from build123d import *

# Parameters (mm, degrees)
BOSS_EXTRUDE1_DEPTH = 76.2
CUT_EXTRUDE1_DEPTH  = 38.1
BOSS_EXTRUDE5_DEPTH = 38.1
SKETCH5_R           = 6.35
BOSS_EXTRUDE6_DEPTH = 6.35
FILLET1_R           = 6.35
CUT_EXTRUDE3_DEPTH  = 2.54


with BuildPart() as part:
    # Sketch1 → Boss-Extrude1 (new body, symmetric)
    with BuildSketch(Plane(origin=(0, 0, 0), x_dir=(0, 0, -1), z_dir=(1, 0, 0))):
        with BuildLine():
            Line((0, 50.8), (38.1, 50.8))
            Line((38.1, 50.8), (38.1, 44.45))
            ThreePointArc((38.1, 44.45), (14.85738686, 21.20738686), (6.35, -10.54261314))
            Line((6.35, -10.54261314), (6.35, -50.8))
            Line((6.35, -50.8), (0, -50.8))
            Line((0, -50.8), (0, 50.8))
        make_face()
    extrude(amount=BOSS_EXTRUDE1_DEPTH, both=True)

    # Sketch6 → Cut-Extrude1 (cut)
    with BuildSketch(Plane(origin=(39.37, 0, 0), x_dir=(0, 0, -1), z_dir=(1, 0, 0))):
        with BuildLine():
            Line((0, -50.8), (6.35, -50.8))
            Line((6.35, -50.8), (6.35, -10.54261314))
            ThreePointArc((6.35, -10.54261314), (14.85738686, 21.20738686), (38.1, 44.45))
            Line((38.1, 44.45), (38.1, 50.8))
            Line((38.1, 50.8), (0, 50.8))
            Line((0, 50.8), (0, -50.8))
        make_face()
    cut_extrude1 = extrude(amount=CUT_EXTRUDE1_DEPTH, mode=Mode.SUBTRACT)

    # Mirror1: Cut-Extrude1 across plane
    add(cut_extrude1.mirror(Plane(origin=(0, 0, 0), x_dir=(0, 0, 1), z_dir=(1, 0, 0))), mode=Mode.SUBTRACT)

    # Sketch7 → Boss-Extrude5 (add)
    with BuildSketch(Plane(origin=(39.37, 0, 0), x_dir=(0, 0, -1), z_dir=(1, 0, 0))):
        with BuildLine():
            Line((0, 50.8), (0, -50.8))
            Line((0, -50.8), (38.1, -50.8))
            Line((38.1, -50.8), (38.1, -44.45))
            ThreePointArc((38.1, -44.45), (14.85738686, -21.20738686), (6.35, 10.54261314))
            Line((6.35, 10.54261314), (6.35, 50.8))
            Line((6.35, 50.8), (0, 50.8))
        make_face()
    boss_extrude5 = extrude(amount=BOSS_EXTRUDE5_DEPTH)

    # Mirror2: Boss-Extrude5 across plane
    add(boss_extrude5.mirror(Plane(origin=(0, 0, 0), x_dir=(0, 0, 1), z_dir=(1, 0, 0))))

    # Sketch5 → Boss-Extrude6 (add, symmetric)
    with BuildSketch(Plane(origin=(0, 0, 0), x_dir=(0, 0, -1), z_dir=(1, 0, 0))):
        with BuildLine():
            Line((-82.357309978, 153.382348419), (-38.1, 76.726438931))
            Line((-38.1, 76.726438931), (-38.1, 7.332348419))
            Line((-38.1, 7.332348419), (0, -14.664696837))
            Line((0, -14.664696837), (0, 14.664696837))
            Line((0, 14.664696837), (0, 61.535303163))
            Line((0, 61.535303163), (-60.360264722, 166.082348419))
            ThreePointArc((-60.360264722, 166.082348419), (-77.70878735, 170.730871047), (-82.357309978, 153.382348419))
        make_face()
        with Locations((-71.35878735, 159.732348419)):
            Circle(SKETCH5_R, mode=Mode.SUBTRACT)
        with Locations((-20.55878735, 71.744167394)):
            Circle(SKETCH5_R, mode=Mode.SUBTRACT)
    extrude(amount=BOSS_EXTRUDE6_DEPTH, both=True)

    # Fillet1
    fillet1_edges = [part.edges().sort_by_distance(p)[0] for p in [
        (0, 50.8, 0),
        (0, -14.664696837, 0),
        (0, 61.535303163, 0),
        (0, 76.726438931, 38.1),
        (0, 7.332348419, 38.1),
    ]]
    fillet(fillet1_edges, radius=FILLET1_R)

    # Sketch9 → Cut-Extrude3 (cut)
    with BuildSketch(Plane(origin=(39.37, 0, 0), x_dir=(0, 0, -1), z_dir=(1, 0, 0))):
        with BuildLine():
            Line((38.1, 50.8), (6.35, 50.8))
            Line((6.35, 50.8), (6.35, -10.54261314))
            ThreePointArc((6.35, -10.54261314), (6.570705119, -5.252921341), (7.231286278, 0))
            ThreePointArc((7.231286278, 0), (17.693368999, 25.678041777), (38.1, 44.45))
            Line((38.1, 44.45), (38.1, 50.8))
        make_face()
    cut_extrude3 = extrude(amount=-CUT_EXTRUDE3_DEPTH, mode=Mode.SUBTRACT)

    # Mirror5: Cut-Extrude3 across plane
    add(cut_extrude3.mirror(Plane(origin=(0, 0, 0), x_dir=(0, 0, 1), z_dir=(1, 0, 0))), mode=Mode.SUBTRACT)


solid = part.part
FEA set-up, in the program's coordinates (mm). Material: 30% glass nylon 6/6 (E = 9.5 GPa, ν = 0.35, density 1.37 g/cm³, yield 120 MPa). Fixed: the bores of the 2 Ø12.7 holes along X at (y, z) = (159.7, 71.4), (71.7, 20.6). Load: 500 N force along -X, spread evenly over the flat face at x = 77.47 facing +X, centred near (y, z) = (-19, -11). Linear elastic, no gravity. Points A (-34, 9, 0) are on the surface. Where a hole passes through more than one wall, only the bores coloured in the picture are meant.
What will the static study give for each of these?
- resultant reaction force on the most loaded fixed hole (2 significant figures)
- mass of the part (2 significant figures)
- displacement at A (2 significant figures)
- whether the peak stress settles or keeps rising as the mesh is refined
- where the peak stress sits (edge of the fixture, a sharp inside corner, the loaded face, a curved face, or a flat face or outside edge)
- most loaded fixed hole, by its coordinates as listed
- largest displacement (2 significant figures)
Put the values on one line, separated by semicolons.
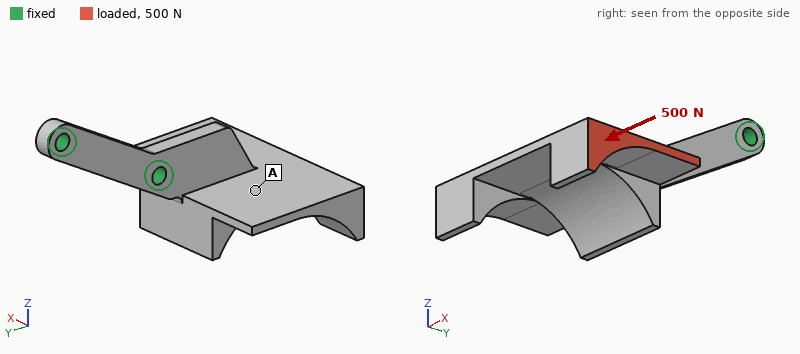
510 N; 380 g; 1.3 mm; keeps rising; edge of the fixture; (71.7, 20.6); 3.3 mm
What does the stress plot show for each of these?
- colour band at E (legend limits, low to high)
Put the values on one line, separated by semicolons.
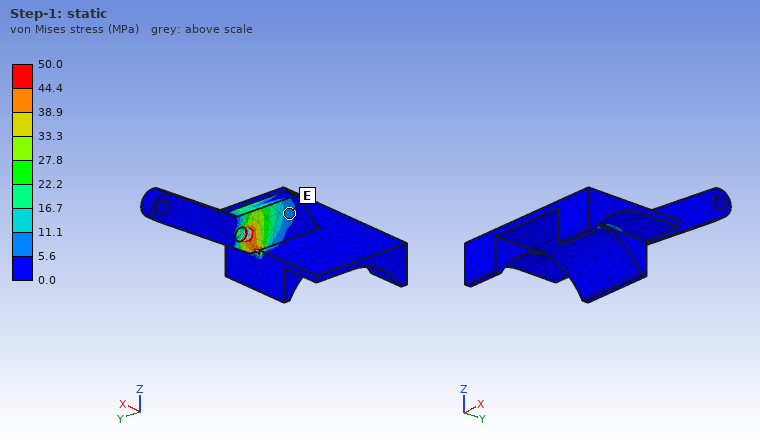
5.6 to 11.1 MPa
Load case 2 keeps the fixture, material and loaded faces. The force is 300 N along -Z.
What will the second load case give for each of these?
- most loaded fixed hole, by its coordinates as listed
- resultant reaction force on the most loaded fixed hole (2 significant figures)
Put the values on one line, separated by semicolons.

(71.7, 20.6); 330 N
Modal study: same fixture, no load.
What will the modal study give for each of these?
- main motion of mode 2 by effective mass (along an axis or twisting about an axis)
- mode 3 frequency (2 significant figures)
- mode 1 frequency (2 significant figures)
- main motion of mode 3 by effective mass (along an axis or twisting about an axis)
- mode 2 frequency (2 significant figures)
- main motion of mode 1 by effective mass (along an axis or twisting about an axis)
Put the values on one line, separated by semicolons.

twisting about Y; 290 Hz; 150 Hz; along Z; 240 Hz; along X
